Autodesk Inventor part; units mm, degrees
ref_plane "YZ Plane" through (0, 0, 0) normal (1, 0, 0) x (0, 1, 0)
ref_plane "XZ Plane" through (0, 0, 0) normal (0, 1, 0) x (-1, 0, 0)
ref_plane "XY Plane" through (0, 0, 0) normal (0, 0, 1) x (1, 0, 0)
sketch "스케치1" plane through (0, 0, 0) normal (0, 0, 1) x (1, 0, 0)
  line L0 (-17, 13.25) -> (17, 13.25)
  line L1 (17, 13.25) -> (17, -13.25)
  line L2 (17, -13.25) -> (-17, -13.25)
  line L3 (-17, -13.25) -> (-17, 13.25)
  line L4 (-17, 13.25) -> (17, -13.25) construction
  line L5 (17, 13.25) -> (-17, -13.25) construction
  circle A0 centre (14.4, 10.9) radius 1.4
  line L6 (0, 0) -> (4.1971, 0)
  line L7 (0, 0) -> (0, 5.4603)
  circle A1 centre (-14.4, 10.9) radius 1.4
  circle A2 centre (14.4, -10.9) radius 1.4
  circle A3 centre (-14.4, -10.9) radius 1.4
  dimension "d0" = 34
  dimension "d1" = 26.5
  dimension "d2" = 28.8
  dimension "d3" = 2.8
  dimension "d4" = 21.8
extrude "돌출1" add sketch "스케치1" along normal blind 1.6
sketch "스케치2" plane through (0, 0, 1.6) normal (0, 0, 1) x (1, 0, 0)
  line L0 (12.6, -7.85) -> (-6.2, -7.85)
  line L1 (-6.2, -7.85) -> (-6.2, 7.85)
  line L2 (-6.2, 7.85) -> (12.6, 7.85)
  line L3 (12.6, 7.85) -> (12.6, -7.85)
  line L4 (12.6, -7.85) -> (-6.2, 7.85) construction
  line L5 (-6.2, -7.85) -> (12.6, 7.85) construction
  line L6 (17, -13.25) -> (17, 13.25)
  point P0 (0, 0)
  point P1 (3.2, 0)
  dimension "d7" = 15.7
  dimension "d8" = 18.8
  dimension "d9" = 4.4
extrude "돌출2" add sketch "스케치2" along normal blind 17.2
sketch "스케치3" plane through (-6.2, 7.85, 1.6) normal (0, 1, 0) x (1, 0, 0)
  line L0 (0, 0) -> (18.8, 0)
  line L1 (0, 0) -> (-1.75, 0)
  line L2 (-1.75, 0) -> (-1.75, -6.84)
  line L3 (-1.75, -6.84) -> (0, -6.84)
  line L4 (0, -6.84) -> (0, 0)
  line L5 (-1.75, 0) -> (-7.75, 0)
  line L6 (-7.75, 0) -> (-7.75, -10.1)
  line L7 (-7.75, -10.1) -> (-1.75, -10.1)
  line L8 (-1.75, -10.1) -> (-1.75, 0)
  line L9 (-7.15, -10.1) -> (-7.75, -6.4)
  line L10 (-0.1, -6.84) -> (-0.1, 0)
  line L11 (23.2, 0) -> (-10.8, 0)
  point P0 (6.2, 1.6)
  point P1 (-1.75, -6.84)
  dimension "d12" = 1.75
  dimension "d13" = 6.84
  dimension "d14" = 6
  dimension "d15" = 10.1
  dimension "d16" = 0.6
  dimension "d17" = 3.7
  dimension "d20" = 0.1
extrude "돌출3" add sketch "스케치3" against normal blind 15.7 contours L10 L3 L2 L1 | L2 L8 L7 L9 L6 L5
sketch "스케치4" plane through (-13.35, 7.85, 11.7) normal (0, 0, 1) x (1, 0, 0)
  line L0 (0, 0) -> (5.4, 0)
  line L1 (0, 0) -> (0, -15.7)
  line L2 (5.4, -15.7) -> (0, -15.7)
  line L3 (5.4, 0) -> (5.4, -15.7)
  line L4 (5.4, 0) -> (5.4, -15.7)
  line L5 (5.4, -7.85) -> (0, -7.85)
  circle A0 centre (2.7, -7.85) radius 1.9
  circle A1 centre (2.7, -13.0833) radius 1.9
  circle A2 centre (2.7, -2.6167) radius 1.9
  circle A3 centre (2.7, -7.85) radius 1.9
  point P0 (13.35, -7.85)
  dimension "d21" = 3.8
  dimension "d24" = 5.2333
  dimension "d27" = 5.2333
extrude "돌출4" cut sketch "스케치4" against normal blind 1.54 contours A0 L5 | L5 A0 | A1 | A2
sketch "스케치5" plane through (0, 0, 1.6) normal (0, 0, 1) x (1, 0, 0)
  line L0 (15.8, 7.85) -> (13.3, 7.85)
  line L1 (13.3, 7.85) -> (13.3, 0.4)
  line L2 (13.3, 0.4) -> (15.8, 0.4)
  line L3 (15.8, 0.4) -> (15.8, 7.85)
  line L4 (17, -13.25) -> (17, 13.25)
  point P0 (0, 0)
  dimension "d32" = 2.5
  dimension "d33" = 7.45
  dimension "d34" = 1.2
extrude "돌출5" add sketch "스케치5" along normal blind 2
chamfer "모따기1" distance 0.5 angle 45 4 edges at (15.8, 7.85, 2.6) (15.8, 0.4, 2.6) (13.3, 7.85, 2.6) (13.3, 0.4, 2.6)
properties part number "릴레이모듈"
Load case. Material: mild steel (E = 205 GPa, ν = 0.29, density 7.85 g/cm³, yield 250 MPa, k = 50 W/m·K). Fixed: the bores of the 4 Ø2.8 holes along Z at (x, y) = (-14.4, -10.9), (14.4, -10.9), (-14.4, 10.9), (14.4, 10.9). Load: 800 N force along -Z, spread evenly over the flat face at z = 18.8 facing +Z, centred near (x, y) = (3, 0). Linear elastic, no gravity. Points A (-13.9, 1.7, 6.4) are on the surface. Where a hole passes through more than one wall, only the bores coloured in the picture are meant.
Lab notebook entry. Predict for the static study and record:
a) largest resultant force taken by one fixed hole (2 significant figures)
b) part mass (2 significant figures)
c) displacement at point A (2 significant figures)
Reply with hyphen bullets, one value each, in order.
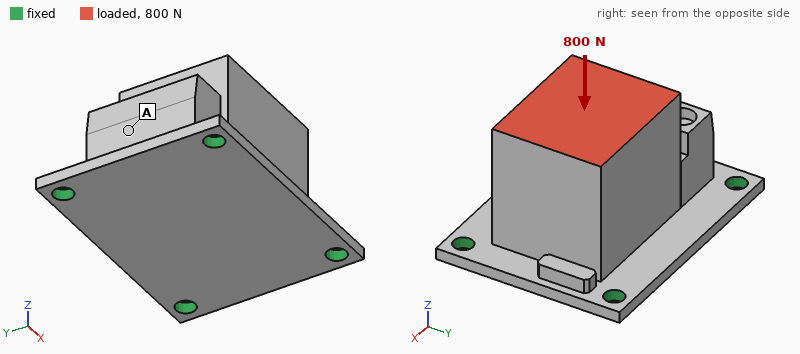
- 280 N
- 59 g
- 6.9 µm
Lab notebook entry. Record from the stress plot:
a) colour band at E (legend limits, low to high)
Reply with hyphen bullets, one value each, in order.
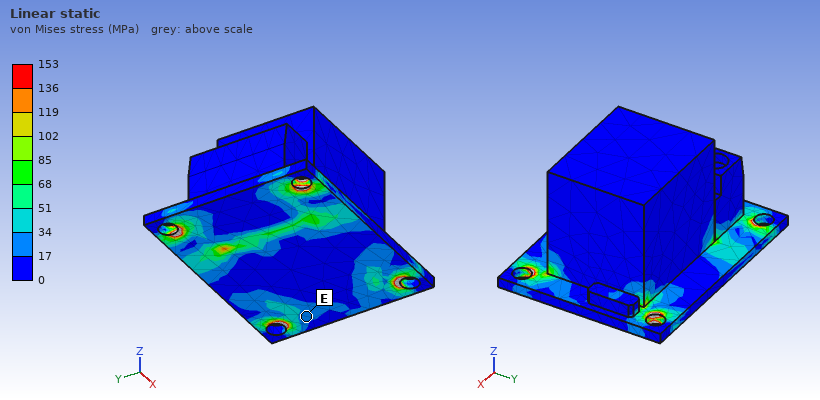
- 17 to 34 MPa
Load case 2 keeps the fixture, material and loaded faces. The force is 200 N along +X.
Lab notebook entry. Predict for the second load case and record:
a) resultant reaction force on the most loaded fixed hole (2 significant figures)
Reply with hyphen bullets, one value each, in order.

- 110 N
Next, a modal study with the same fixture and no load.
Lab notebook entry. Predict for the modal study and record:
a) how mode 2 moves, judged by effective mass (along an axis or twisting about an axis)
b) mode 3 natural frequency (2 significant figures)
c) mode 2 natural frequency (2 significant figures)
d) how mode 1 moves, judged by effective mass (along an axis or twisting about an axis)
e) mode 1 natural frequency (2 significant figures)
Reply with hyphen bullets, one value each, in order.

- along Y
- 9500 Hz
- 7400 Hz
- along Z
- 5300 Hz
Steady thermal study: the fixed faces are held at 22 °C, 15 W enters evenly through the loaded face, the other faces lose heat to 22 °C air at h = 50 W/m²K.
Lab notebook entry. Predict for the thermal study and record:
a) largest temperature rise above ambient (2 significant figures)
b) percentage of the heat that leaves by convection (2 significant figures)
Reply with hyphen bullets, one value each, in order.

- 42 K
- 25 %
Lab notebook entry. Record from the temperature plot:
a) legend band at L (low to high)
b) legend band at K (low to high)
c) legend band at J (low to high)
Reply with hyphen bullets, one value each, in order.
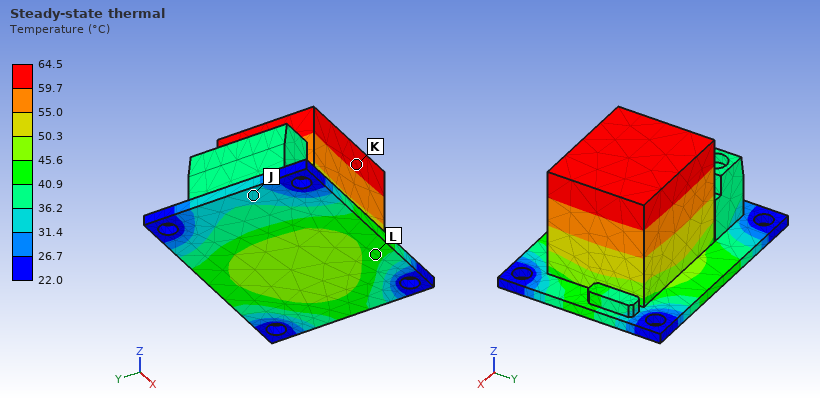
- 40.9 to 45.6 °C
- 59.7 to 64.5 °C
- 31.4 to 36.2 °C
